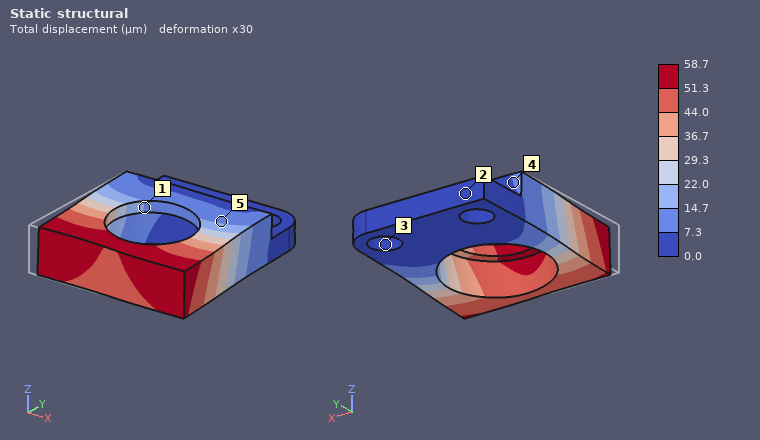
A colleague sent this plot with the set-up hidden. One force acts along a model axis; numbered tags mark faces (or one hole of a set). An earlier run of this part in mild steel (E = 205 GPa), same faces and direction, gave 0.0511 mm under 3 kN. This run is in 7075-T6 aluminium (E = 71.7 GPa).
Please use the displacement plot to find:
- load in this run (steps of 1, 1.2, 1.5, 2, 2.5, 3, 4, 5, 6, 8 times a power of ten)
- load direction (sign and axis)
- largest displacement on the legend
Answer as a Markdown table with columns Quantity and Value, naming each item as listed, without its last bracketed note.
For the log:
| Quantity | Value |
|---|---|
| load in this run | 1.2 kN |
| load direction | +X |
| largest displacement on the legend | 58.7 µm |
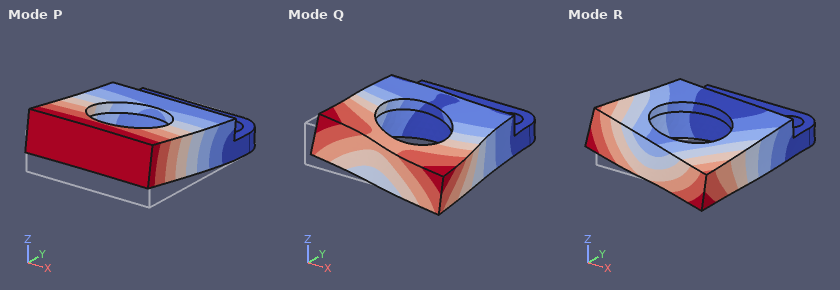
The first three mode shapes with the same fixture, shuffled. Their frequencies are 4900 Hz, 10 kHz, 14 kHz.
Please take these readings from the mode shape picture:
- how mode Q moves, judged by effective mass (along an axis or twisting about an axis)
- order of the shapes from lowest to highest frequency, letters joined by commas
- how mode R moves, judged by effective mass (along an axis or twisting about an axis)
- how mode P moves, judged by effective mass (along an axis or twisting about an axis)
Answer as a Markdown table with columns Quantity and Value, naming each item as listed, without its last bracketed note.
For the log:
| Quantity | Value |
|---|---|
| how mode Q moves, judged by effective mass | along X |
| order of the shapes from lowest to highest frequency, letters joined by commas | P, R, Q |
| how mode R moves, judged by effective mass | along X |
| how mode P moves, judged by effective mass | along Z |
